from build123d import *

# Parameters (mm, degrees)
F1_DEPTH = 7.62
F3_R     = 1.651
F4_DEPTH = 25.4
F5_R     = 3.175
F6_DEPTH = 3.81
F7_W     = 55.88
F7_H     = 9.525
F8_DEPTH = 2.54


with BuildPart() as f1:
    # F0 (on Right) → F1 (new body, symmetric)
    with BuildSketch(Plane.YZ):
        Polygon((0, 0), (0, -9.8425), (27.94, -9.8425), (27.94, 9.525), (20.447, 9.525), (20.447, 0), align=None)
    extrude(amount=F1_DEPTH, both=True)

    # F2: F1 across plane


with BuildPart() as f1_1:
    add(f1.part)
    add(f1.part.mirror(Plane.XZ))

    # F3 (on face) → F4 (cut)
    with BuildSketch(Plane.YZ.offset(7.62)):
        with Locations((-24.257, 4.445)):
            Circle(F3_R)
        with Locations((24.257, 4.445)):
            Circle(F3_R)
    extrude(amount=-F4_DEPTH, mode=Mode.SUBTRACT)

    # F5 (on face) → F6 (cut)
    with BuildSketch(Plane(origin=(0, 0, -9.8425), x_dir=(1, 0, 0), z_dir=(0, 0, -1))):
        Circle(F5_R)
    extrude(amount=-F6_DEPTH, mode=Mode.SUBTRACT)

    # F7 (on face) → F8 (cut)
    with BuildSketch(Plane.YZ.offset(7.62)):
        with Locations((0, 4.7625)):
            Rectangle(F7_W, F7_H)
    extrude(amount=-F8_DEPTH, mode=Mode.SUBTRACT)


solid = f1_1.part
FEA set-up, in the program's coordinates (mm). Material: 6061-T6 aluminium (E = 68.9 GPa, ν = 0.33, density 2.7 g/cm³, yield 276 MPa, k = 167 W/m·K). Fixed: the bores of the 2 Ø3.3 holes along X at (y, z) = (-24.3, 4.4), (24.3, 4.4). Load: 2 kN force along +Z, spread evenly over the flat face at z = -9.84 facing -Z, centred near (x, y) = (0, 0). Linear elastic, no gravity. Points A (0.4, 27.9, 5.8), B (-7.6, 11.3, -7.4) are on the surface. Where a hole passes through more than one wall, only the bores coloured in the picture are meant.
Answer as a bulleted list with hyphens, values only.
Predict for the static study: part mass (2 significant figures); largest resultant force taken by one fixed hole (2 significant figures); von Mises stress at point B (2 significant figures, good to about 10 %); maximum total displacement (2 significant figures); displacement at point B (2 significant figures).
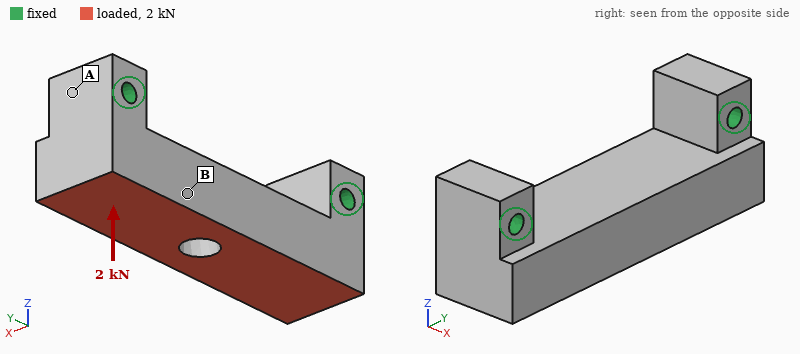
- 27 g
- 1.2 kN
- 11 MPa
- 15 µm
- 8.7 µm
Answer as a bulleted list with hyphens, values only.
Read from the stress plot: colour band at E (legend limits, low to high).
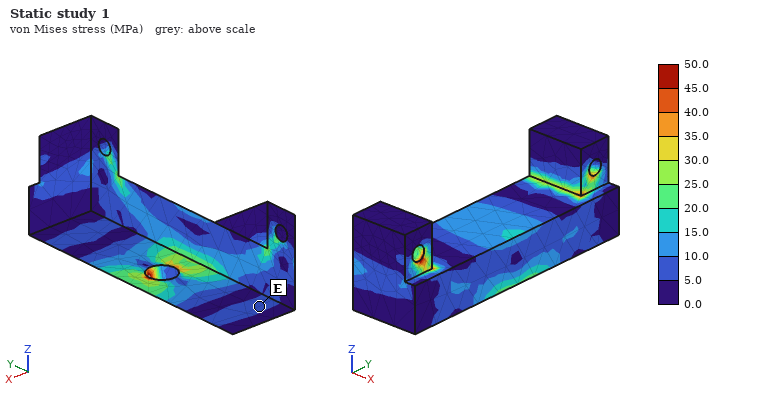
- 5.0 to 10.0 MPa
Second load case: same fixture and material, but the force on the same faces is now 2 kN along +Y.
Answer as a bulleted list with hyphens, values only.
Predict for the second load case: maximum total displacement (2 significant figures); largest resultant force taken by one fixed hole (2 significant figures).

- 9.3 µm
- 1.1 kN
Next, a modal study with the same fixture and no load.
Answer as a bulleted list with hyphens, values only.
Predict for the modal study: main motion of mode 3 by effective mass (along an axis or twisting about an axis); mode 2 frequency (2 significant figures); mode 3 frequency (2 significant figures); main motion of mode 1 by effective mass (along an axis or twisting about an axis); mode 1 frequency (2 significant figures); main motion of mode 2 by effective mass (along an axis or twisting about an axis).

- along Y
- 15 kHz
- 18 kHz
- along X
- 13 kHz
- along Z
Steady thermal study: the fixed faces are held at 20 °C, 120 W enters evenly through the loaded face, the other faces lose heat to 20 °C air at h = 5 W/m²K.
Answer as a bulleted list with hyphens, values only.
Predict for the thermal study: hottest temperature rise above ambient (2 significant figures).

- 48 K
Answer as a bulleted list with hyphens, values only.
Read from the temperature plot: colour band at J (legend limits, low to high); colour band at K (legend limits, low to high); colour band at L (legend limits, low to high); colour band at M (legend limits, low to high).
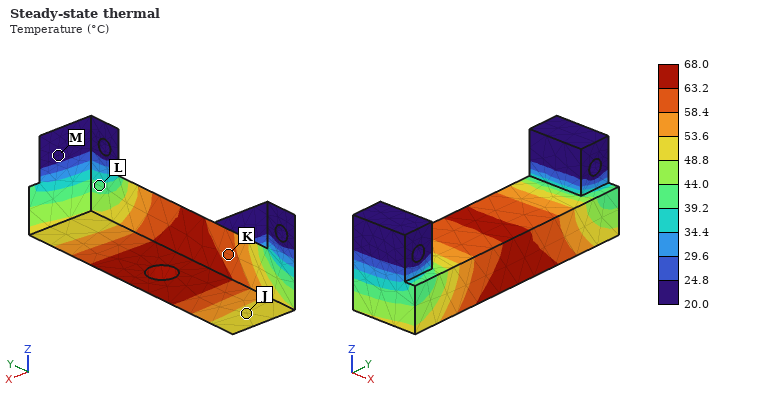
- 48.8 to 53.6 °C
- 58.4 to 63.2 °C
- 39.2 to 44.0 °C
- 20.0 to 24.8 °C
